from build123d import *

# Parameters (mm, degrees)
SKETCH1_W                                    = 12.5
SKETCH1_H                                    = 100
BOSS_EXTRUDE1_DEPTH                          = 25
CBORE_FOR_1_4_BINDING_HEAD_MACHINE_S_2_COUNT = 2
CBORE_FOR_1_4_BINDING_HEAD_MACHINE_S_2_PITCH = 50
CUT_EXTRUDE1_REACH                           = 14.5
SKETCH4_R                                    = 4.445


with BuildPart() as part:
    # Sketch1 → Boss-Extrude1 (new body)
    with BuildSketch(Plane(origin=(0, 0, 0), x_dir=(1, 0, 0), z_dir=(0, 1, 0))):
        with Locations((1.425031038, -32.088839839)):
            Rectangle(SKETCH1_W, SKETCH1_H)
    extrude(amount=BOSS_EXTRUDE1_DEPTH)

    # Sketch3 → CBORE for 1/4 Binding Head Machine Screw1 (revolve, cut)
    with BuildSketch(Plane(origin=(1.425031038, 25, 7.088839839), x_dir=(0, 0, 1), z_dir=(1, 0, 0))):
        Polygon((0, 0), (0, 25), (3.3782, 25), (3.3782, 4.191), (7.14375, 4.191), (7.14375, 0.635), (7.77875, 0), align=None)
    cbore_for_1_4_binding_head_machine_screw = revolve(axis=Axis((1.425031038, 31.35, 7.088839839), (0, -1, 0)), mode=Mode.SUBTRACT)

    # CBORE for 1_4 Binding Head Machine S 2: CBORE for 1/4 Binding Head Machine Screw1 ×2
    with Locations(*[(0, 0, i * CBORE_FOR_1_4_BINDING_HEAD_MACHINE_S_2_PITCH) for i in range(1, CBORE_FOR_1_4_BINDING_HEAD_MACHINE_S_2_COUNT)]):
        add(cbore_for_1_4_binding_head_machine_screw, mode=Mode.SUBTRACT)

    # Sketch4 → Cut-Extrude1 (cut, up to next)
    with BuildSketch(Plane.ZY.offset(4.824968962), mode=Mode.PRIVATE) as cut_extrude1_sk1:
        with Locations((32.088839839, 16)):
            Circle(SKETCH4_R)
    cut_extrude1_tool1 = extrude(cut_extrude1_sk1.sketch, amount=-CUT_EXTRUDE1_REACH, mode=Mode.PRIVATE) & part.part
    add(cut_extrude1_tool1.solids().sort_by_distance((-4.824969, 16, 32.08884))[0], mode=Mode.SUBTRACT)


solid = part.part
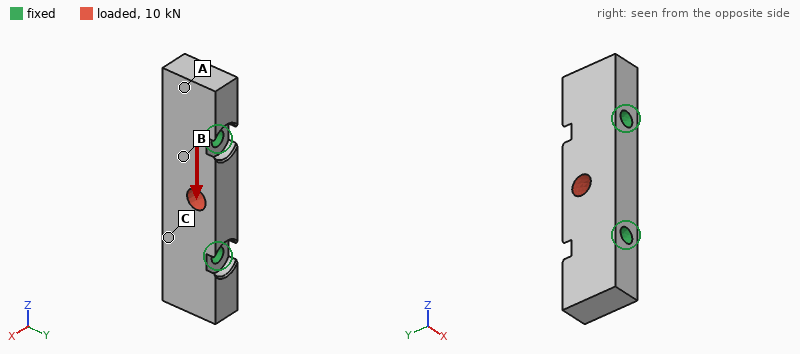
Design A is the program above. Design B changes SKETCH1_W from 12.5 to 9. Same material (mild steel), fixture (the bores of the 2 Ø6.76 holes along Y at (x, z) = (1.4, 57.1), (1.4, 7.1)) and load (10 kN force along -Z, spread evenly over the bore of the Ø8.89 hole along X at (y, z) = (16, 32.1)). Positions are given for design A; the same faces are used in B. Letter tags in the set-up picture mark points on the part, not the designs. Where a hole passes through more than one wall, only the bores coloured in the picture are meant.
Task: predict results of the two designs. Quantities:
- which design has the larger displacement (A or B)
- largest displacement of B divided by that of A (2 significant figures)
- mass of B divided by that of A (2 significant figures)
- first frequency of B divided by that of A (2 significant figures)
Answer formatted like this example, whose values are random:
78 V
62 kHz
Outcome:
B
1.4
0.70
0.87
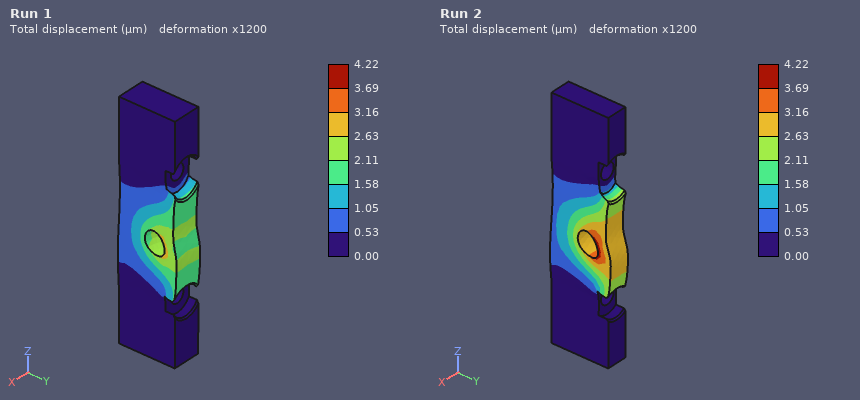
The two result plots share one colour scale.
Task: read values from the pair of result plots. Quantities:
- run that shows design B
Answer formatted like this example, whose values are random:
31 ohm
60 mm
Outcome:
Run 2
